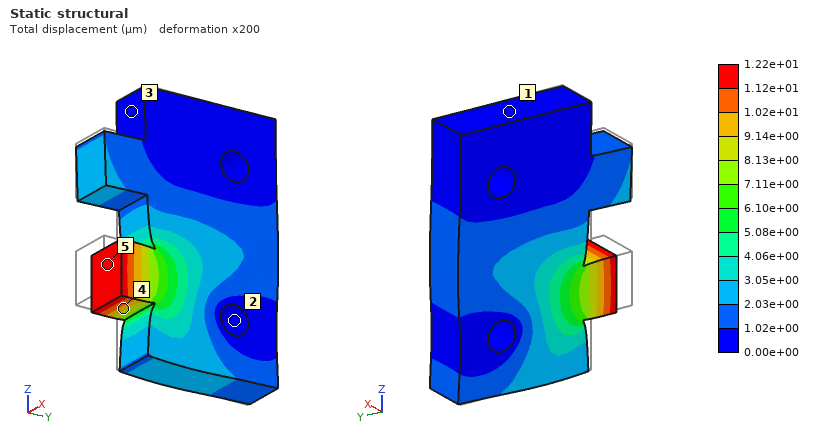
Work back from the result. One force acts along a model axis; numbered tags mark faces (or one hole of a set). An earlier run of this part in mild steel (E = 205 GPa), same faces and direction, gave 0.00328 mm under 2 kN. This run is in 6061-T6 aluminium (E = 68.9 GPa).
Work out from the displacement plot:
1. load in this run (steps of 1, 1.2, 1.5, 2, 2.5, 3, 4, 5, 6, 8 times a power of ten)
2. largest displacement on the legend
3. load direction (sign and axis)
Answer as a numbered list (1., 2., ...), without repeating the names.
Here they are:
1. 2.5 kN
2. 1.22e+01 µm
3. +Y
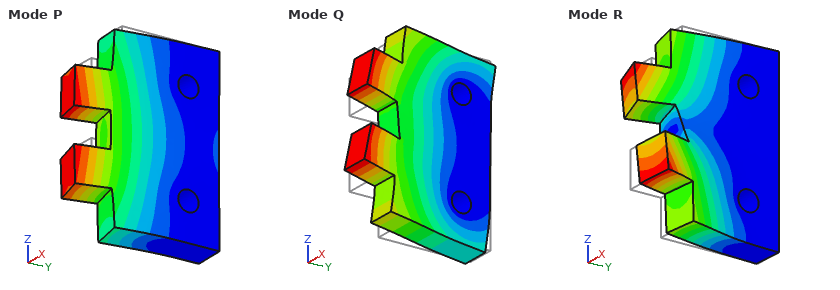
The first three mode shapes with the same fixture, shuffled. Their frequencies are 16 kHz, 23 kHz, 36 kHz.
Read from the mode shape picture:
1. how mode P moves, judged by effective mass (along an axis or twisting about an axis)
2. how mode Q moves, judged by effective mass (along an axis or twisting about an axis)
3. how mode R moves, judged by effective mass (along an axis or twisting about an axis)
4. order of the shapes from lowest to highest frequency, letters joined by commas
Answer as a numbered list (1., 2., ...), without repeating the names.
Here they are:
1. along X
2. along Z
3. twisting about Y
4. P, R, Q
